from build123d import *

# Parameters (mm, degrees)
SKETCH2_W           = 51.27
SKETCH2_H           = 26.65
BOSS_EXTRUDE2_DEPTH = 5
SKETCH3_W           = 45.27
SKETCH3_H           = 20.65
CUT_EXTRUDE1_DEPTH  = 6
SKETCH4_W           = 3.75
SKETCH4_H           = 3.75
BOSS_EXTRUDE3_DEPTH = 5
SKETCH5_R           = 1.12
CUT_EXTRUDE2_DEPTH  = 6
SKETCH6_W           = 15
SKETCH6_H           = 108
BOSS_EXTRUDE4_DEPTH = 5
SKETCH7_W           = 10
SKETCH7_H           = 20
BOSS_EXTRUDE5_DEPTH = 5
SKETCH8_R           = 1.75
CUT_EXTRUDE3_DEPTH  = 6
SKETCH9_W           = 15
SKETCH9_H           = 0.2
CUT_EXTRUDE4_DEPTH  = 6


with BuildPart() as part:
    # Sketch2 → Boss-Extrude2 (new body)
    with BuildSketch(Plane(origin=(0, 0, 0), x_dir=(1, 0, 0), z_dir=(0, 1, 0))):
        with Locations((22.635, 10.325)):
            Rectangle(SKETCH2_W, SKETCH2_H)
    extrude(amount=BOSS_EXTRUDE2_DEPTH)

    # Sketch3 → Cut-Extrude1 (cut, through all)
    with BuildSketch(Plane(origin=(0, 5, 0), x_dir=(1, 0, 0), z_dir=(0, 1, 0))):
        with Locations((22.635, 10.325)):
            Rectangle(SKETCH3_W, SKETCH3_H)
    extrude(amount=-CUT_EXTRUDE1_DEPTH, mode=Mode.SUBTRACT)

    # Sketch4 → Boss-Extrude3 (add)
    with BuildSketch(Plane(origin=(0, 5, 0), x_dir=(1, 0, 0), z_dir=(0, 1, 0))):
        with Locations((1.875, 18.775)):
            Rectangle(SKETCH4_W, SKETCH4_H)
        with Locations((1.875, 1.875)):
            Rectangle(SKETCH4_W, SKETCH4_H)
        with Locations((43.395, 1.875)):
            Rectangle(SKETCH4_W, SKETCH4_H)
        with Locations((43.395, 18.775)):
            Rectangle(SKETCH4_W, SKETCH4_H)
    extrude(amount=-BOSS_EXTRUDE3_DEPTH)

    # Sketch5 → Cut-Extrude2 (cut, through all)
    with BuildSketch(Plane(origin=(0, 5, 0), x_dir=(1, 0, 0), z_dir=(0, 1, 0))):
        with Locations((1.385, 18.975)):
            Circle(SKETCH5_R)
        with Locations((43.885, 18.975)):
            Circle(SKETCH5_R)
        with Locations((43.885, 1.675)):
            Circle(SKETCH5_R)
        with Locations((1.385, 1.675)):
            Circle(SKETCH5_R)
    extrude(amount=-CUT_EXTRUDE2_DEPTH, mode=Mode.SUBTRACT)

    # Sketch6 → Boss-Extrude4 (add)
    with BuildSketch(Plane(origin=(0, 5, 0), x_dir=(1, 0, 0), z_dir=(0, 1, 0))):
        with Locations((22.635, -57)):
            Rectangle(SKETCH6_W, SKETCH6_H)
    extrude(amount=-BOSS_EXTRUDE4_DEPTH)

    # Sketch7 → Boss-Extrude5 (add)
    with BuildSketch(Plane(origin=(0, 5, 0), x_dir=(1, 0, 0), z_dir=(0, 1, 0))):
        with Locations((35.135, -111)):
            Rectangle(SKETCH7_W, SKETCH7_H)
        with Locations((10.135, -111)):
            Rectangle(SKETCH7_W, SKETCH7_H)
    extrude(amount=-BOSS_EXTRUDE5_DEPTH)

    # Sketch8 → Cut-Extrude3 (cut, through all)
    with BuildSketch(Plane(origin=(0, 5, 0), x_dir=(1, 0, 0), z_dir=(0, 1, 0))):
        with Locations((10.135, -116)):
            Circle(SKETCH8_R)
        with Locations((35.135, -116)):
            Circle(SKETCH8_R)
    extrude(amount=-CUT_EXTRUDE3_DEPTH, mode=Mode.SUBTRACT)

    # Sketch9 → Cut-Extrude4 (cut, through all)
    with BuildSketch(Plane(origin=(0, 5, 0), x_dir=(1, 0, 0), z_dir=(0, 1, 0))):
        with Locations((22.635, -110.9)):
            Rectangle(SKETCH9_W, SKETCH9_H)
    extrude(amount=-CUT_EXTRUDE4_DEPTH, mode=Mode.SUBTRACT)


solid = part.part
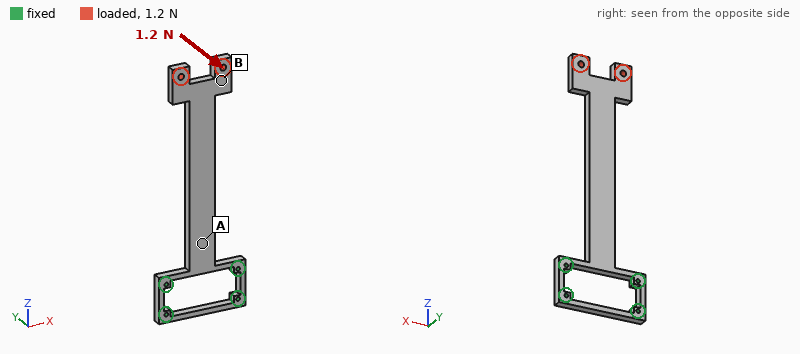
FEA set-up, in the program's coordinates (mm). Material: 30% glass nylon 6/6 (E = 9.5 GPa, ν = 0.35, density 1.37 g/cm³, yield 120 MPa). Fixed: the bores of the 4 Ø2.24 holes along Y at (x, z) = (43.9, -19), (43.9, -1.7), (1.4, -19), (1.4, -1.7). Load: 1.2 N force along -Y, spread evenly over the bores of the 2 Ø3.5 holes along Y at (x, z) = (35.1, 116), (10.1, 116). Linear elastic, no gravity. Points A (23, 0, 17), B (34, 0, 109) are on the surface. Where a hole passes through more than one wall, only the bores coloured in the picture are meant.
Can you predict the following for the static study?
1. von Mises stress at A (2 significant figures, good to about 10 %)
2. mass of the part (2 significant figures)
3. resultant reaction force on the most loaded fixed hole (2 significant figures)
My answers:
1.9 MPa
17 g
0.80 N
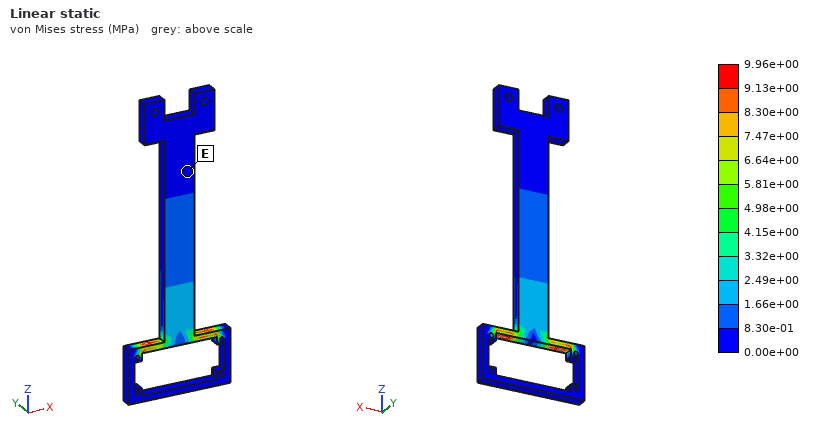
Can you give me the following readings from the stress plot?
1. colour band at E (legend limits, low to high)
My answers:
0.00e+00 to 8.30e-01 MPa
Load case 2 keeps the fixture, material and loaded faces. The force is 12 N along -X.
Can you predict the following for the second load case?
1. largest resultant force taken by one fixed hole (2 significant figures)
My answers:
58 N
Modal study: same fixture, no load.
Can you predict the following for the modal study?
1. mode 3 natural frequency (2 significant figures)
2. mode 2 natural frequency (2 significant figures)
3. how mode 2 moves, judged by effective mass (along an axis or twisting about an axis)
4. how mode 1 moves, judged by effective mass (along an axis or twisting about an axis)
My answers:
640 Hz
190 Hz
along X
along Y
